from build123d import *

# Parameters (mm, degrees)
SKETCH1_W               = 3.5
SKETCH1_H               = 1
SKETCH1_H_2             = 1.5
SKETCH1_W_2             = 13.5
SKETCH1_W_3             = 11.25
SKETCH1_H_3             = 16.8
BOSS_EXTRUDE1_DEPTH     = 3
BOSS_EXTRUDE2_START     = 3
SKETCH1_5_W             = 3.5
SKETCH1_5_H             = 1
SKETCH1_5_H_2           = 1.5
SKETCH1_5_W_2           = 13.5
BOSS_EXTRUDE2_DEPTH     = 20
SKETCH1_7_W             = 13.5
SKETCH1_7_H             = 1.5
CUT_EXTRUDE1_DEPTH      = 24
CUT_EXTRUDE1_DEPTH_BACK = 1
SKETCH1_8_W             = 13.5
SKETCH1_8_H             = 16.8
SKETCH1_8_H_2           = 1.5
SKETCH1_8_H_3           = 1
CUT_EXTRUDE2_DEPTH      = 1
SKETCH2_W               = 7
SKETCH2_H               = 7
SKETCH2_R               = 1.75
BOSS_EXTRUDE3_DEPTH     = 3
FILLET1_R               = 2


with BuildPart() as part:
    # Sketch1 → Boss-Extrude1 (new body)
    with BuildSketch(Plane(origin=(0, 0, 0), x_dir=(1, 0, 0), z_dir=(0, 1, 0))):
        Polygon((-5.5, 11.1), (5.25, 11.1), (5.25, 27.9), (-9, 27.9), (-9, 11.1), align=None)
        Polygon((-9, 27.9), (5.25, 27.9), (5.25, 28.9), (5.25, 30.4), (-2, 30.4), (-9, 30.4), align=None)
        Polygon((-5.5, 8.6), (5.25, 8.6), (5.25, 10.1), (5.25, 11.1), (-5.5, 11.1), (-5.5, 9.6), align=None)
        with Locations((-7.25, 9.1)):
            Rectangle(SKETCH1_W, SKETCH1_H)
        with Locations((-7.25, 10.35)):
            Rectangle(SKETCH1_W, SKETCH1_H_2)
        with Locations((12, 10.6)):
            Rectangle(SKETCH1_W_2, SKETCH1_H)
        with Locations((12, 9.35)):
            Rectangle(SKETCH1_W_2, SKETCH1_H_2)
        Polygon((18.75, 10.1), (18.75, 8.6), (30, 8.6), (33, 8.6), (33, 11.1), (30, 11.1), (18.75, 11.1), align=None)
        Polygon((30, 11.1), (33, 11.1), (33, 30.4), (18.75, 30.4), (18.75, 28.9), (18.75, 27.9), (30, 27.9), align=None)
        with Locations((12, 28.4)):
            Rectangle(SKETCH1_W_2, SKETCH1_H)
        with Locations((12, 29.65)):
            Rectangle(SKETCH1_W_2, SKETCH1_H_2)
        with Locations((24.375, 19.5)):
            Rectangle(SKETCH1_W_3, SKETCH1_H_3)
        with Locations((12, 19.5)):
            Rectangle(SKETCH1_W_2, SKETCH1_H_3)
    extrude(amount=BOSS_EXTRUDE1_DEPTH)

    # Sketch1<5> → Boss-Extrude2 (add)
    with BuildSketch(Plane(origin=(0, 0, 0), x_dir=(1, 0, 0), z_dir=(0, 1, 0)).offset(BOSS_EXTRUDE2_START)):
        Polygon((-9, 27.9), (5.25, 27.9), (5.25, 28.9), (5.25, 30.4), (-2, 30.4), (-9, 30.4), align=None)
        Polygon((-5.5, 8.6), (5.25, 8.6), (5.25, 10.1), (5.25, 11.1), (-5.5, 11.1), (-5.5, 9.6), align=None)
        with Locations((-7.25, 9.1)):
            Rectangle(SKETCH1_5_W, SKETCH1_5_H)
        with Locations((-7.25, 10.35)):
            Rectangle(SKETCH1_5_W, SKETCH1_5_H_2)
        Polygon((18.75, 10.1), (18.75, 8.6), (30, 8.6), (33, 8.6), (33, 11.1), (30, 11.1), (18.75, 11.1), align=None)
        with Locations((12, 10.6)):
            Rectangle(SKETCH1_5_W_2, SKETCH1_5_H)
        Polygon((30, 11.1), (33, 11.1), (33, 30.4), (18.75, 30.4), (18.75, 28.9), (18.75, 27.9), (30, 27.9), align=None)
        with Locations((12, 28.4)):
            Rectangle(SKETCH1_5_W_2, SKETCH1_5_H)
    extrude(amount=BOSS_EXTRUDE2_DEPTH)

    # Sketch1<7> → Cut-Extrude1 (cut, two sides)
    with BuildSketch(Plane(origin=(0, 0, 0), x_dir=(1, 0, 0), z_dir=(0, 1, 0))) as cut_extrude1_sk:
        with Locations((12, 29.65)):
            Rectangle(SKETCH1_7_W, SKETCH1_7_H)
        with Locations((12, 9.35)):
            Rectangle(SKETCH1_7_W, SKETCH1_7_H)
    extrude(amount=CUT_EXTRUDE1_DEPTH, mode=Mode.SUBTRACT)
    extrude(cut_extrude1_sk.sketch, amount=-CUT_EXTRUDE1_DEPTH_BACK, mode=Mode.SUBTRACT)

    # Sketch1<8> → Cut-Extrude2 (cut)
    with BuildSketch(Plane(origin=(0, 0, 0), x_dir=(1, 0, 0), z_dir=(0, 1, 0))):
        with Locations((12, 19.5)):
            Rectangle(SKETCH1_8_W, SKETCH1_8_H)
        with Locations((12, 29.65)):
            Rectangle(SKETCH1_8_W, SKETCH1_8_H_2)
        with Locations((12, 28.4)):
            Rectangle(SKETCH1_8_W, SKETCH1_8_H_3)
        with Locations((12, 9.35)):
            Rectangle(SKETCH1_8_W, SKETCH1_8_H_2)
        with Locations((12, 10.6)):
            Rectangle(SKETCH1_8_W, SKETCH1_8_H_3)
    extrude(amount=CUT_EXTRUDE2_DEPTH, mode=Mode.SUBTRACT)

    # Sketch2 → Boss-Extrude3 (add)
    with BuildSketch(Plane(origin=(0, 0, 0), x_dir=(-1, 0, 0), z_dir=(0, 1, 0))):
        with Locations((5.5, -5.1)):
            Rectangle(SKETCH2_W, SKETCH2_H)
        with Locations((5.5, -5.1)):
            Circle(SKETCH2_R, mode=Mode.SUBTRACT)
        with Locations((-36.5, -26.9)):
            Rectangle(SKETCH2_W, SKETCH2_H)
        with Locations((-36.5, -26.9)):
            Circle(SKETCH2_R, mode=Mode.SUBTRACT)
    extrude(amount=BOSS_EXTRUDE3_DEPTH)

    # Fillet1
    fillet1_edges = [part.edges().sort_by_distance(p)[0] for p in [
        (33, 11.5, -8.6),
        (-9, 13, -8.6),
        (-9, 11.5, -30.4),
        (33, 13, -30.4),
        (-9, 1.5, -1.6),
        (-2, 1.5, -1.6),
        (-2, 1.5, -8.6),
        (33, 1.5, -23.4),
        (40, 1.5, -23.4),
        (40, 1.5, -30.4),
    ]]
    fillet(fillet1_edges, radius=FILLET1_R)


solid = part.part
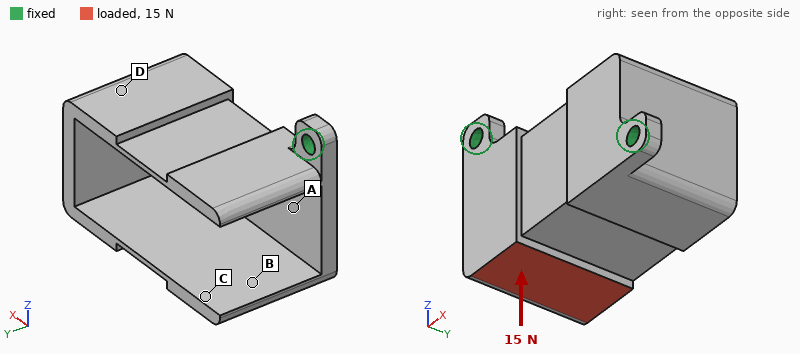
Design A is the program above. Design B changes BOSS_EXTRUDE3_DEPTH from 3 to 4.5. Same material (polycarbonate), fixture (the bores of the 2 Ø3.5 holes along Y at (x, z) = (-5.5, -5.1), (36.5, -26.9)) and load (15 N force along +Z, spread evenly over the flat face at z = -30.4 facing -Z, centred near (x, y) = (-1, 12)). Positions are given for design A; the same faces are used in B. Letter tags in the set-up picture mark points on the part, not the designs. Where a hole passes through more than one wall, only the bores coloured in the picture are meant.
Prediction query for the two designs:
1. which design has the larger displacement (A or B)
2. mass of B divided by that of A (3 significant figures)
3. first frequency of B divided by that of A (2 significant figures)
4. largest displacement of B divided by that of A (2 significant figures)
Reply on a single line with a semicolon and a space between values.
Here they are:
A; 1.02; 1.3; 0.88
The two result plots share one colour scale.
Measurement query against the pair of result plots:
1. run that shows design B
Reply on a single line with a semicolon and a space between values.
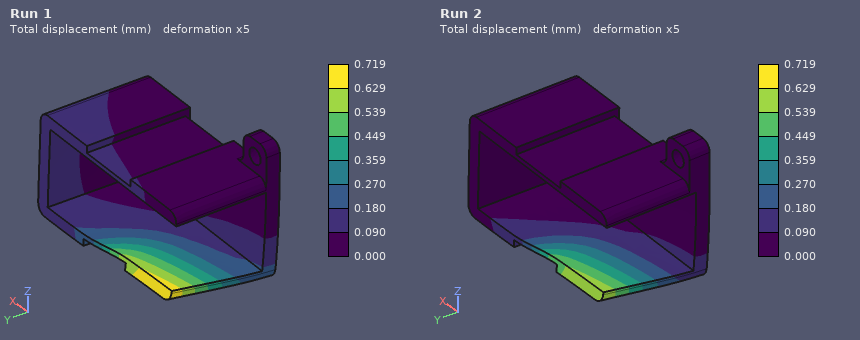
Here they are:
Run 2
